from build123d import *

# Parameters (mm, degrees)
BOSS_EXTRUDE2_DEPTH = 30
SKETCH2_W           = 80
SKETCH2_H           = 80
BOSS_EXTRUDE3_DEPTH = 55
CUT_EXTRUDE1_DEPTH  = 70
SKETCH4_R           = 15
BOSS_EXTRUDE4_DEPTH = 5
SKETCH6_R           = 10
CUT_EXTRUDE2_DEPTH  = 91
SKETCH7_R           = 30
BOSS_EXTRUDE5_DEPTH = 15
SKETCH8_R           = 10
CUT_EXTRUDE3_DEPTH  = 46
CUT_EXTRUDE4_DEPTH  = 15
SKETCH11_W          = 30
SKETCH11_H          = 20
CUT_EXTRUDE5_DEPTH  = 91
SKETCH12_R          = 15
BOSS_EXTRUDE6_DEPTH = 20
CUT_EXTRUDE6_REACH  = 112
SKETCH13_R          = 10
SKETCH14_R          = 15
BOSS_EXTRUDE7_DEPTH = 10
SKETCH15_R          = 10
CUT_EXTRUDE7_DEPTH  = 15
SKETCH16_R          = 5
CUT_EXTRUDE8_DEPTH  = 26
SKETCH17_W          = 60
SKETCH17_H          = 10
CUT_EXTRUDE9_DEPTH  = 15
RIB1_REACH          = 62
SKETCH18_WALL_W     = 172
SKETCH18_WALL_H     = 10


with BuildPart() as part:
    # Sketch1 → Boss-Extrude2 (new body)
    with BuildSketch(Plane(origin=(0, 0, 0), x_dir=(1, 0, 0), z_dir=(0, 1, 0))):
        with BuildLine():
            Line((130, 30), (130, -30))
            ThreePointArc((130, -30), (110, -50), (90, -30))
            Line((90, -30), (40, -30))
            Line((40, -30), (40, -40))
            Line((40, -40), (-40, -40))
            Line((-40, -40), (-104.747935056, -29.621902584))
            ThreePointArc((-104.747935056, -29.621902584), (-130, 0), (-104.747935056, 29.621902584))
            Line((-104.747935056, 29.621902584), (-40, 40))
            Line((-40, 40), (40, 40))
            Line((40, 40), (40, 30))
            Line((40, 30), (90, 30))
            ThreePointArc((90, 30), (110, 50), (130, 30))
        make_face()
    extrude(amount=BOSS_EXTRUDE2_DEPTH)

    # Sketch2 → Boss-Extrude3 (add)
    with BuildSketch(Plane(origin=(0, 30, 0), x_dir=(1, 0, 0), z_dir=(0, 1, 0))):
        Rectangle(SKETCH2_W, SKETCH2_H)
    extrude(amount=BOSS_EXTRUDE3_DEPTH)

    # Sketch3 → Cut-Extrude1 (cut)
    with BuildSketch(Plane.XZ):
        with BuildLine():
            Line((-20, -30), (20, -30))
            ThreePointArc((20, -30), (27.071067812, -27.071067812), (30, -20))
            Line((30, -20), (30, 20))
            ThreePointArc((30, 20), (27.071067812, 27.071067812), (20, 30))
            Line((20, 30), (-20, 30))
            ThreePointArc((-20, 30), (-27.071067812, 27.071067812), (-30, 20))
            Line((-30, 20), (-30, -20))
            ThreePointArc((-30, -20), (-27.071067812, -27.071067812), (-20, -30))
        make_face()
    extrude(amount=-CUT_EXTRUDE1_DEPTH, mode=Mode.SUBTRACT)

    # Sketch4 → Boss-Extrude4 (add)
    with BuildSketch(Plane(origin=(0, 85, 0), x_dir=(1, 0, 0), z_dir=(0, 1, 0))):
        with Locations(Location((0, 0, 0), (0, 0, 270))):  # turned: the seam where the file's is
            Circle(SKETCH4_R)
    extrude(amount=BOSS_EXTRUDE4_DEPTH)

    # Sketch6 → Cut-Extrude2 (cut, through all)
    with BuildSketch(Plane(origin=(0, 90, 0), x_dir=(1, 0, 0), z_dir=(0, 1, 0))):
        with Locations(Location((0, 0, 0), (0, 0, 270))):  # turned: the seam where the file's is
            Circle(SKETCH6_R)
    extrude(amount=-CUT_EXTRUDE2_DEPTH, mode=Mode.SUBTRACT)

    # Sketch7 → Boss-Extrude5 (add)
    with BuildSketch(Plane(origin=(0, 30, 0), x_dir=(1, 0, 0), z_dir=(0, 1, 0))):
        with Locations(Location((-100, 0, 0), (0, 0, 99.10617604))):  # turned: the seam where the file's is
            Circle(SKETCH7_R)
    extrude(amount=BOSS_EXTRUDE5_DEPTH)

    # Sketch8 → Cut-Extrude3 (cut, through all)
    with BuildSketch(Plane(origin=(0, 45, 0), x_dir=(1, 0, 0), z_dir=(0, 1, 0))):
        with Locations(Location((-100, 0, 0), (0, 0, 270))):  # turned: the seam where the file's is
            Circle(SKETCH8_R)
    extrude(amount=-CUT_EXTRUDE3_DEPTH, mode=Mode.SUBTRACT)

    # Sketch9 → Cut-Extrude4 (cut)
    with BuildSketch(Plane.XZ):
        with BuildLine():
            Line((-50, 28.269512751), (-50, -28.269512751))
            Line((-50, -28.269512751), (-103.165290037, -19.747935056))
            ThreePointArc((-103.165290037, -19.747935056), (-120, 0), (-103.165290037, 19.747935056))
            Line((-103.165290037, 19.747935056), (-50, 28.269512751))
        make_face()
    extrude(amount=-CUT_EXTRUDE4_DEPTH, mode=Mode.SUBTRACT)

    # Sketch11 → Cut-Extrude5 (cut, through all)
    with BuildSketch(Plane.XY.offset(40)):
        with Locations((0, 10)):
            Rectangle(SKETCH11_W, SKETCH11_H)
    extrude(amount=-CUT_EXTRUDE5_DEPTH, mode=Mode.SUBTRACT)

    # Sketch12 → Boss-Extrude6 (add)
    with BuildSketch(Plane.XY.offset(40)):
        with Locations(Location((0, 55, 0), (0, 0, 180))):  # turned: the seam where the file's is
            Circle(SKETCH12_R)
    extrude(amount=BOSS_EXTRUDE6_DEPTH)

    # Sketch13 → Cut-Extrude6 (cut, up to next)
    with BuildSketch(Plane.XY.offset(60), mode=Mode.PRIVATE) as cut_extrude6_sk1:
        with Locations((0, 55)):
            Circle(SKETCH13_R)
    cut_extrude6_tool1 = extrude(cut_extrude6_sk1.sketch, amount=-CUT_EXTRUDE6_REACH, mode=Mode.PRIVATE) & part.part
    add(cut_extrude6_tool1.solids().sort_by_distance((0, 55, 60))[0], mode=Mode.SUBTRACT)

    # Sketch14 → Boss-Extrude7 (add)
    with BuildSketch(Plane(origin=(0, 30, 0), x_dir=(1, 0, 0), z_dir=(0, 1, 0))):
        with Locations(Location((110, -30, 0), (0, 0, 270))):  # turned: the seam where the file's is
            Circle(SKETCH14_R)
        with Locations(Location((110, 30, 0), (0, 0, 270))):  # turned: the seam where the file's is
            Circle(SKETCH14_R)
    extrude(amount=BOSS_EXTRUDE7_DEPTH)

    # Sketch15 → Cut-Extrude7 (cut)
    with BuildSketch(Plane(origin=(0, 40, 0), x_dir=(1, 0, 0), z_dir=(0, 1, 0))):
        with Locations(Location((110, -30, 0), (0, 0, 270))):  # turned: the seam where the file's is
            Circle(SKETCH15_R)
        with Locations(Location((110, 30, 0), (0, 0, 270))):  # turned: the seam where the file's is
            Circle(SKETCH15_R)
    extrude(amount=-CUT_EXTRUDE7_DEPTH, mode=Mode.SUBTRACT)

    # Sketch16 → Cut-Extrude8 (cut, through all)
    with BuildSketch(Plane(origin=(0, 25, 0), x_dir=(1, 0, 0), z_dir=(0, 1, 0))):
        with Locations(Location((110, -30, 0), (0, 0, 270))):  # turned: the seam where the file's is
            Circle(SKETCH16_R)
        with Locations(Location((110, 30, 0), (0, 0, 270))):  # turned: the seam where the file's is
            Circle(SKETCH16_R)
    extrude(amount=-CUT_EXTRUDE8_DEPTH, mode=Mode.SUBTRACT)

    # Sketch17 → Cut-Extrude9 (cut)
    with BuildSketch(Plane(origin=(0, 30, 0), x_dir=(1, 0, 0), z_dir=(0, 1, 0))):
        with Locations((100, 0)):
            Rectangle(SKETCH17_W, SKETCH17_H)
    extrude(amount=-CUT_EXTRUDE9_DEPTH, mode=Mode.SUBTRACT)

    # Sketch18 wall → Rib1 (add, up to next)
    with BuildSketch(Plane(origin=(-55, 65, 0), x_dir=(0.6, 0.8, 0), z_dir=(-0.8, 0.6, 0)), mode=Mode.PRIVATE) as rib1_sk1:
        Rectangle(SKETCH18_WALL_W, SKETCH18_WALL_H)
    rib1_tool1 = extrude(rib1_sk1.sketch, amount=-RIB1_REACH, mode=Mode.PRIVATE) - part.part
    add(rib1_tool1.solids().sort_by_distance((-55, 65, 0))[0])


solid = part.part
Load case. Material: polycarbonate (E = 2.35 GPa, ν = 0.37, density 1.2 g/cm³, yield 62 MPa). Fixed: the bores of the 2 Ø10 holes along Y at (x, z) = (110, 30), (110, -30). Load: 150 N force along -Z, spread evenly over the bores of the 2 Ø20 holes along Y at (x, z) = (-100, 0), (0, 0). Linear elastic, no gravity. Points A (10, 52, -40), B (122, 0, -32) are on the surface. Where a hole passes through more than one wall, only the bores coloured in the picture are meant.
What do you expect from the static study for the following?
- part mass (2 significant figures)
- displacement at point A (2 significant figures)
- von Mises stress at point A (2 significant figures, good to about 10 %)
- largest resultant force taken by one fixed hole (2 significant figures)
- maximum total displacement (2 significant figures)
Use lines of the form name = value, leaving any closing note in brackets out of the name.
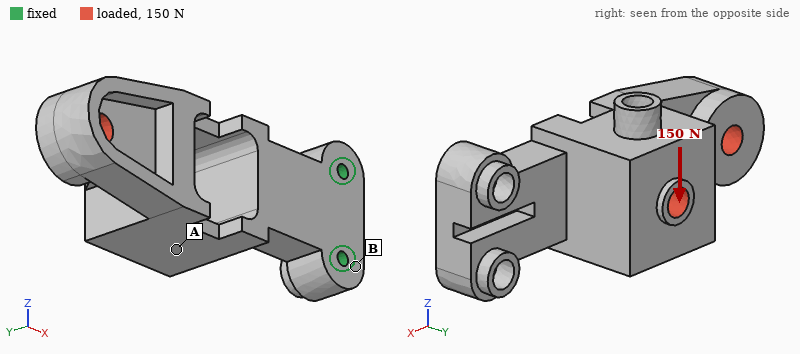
part mass = 780 g
displacement at point A = 0.20 mm
von Mises stress at point A = 0.47 MPa
largest resultant force taken by one fixed hole = 430 N
maximum total displacement = 0.55 mm
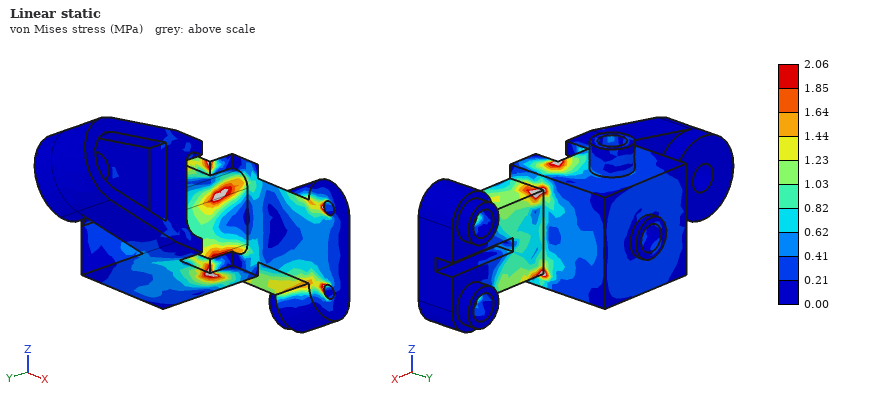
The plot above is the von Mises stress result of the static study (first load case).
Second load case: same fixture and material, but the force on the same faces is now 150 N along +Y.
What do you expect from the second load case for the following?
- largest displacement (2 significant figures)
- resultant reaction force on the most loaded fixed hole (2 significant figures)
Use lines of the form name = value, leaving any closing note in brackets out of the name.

largest displacement = 1.8 mm
resultant reaction force on the most loaded fixed hole = 99 N
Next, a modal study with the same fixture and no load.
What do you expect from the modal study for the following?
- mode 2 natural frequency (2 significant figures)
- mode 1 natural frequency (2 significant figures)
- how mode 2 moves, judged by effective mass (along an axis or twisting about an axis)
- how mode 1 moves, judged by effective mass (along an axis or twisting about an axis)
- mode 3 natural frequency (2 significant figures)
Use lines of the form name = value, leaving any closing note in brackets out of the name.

mode 2 natural frequency = 150 Hz
mode 1 natural frequency = 89 Hz
how mode 2 moves, judged by effective mass = along Z
how mode 1 moves, judged by effective mass = along Y
mode 3 natural frequency = 310 Hz
